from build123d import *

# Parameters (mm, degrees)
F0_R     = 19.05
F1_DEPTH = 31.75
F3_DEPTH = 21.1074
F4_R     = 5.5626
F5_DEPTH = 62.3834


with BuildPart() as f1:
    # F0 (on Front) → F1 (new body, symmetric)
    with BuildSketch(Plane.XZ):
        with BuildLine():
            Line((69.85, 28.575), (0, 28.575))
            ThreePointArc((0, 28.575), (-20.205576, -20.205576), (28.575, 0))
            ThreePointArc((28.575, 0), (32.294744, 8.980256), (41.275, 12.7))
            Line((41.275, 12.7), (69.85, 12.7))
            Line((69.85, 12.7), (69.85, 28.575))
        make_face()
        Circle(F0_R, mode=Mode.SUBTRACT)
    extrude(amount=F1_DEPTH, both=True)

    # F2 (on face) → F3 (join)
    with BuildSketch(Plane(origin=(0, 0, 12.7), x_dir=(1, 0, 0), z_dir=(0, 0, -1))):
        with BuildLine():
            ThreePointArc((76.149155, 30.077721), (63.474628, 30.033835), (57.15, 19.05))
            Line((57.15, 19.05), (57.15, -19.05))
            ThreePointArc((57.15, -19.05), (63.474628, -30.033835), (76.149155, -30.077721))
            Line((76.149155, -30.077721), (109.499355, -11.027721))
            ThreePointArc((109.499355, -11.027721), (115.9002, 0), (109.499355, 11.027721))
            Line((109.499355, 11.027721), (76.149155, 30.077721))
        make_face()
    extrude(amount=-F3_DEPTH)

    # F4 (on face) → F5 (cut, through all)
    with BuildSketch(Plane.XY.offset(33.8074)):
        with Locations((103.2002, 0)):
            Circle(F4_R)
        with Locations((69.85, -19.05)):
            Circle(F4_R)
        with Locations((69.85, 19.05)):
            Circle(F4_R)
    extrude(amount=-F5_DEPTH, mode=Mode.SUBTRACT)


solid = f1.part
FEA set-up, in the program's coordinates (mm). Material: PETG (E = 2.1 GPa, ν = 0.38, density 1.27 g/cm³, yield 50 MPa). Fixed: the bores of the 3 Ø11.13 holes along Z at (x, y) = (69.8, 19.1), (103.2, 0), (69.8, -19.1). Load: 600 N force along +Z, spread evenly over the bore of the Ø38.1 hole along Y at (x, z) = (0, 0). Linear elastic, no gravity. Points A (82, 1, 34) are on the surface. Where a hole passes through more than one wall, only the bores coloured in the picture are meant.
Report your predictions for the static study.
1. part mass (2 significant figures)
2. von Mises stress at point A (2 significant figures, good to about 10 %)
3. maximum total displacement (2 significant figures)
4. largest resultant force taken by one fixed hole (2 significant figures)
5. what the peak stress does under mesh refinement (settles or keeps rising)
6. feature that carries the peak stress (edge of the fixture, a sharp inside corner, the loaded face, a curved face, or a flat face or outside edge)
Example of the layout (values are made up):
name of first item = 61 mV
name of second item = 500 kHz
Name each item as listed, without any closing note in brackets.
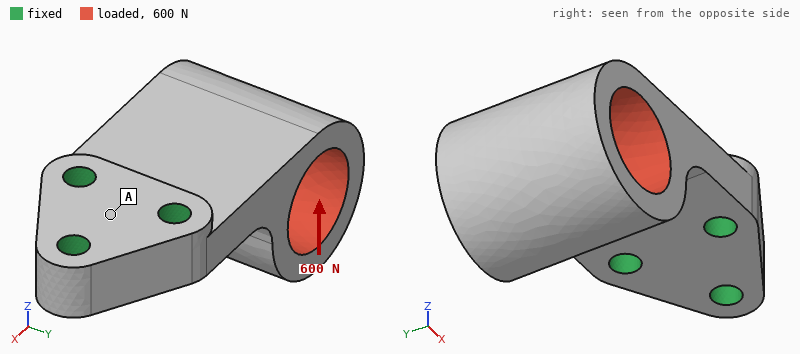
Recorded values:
part mass = 230 g
von Mises stress at point A = 1.7 MPa
maximum total displacement = 2.0 mm
largest resultant force taken by one fixed hole = 370 N
what the peak stress does under mesh refinement = keeps rising
feature that carries the peak stress = edge of the fixture
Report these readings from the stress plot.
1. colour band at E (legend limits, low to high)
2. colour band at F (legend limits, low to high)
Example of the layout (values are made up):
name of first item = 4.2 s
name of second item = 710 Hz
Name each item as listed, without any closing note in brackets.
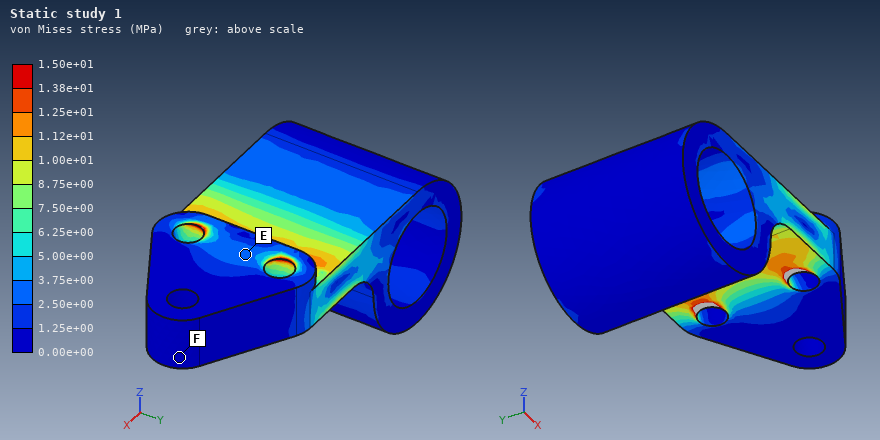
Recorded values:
colour band at E = 2.50e+00 to 3.75e+00 MPa
colour band at F = 0.00e+00 to 1.25e+00 MPa
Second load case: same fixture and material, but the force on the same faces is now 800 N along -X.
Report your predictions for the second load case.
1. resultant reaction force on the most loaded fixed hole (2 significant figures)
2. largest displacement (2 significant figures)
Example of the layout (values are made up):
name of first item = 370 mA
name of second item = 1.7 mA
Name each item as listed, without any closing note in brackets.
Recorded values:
resultant reaction force on the most loaded fixed hole = 380 N
largest displacement = 1.2 mm
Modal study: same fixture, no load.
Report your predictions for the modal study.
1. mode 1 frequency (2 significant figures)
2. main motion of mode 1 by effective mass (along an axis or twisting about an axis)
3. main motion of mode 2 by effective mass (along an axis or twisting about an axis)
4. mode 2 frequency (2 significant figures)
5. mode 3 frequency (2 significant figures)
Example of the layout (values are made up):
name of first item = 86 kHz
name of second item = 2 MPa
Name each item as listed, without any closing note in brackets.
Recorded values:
mode 1 frequency = 270 Hz
main motion of mode 1 by effective mass = along Z
main motion of mode 2 by effective mass = along Y
mode 2 frequency = 660 Hz
mode 3 frequency = 1100 Hz
